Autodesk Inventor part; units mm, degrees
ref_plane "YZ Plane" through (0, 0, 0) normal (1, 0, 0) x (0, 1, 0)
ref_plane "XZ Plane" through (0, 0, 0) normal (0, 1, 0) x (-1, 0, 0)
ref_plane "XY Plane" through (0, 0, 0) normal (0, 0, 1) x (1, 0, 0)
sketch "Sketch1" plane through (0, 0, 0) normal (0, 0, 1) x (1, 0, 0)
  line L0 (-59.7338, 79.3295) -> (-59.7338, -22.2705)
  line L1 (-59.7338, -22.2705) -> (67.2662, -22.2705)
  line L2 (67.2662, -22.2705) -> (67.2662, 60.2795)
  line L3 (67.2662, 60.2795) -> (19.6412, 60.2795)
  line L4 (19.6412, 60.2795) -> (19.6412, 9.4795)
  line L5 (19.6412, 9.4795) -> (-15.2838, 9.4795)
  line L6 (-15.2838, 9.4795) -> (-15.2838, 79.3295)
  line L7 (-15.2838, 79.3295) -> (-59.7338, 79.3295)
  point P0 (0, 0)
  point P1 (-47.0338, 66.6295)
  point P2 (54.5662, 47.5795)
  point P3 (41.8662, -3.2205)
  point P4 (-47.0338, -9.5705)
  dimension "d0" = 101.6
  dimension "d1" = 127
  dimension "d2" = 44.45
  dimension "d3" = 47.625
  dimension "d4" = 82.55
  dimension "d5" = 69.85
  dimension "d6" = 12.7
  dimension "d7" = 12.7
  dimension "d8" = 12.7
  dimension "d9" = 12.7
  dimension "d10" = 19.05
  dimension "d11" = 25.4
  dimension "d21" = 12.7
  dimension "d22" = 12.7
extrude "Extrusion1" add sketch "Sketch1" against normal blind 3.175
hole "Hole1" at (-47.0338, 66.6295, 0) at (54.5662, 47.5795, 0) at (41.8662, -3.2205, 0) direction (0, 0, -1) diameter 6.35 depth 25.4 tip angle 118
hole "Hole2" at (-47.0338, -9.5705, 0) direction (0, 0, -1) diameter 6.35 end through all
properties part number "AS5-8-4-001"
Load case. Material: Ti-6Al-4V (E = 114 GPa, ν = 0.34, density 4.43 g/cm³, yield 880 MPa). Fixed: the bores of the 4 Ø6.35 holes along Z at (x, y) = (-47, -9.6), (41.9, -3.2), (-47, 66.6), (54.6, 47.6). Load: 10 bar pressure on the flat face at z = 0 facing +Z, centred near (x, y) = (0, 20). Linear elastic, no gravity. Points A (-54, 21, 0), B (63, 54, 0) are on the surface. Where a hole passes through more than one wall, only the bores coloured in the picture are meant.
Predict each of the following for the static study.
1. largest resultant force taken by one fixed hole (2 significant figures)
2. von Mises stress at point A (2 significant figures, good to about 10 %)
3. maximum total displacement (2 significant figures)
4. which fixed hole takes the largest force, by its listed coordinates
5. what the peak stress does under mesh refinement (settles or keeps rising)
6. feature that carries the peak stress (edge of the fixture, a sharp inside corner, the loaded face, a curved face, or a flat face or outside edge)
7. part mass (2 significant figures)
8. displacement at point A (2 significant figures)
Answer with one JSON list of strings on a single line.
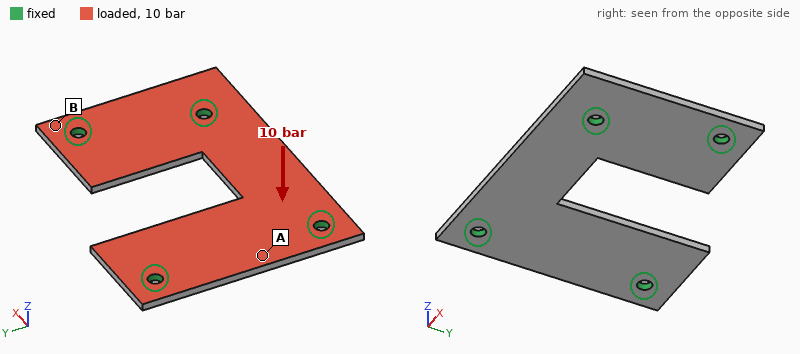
["3.0 kN", "120 MPa", "0.83 mm", "(41.9, -3.2)", "keeps rising", "edge of the fixture", "130 g", "0.21 mm"]
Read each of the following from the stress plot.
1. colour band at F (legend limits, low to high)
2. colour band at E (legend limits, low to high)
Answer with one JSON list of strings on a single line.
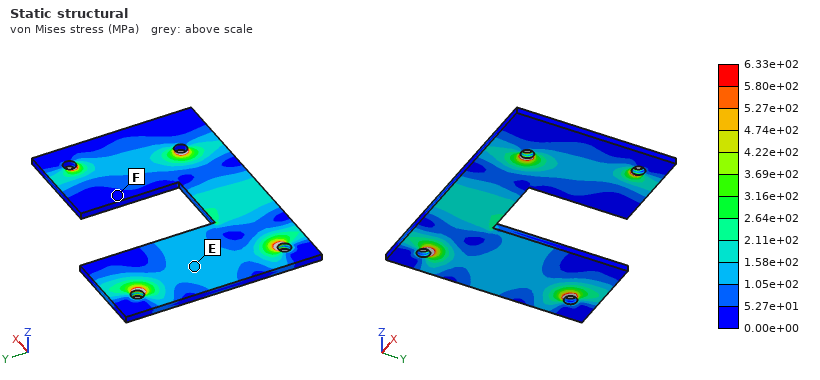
["0.00e+00 to 5.27e+01 MPa", "1.05e+02 to 1.58e+02 MPa"]
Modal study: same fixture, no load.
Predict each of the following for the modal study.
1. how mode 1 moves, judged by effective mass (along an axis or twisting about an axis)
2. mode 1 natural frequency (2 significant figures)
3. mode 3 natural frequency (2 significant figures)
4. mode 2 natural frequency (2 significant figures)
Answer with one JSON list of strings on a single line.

["along Z", "2000 Hz", "2700 Hz", "2500 Hz"]
